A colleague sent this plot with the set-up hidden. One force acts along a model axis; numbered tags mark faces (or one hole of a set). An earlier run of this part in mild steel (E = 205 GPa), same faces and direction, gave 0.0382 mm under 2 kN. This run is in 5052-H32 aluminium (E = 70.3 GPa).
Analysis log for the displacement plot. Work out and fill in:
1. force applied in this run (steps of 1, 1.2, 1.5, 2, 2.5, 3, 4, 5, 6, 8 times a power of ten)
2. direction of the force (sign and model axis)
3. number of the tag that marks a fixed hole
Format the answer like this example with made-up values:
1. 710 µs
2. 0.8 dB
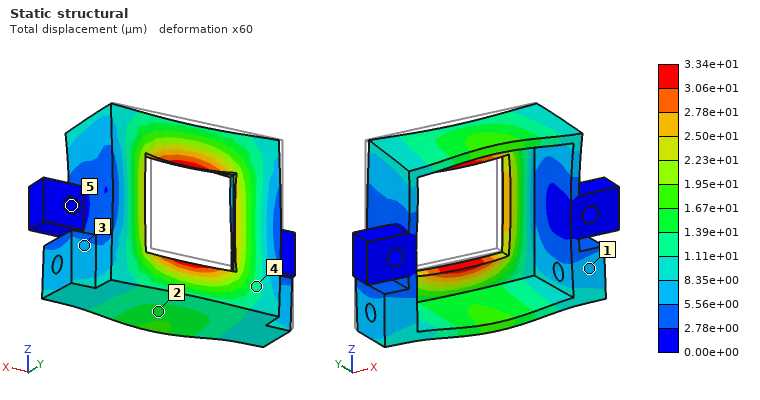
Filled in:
1. 600 N
2. -Y
3. 5
